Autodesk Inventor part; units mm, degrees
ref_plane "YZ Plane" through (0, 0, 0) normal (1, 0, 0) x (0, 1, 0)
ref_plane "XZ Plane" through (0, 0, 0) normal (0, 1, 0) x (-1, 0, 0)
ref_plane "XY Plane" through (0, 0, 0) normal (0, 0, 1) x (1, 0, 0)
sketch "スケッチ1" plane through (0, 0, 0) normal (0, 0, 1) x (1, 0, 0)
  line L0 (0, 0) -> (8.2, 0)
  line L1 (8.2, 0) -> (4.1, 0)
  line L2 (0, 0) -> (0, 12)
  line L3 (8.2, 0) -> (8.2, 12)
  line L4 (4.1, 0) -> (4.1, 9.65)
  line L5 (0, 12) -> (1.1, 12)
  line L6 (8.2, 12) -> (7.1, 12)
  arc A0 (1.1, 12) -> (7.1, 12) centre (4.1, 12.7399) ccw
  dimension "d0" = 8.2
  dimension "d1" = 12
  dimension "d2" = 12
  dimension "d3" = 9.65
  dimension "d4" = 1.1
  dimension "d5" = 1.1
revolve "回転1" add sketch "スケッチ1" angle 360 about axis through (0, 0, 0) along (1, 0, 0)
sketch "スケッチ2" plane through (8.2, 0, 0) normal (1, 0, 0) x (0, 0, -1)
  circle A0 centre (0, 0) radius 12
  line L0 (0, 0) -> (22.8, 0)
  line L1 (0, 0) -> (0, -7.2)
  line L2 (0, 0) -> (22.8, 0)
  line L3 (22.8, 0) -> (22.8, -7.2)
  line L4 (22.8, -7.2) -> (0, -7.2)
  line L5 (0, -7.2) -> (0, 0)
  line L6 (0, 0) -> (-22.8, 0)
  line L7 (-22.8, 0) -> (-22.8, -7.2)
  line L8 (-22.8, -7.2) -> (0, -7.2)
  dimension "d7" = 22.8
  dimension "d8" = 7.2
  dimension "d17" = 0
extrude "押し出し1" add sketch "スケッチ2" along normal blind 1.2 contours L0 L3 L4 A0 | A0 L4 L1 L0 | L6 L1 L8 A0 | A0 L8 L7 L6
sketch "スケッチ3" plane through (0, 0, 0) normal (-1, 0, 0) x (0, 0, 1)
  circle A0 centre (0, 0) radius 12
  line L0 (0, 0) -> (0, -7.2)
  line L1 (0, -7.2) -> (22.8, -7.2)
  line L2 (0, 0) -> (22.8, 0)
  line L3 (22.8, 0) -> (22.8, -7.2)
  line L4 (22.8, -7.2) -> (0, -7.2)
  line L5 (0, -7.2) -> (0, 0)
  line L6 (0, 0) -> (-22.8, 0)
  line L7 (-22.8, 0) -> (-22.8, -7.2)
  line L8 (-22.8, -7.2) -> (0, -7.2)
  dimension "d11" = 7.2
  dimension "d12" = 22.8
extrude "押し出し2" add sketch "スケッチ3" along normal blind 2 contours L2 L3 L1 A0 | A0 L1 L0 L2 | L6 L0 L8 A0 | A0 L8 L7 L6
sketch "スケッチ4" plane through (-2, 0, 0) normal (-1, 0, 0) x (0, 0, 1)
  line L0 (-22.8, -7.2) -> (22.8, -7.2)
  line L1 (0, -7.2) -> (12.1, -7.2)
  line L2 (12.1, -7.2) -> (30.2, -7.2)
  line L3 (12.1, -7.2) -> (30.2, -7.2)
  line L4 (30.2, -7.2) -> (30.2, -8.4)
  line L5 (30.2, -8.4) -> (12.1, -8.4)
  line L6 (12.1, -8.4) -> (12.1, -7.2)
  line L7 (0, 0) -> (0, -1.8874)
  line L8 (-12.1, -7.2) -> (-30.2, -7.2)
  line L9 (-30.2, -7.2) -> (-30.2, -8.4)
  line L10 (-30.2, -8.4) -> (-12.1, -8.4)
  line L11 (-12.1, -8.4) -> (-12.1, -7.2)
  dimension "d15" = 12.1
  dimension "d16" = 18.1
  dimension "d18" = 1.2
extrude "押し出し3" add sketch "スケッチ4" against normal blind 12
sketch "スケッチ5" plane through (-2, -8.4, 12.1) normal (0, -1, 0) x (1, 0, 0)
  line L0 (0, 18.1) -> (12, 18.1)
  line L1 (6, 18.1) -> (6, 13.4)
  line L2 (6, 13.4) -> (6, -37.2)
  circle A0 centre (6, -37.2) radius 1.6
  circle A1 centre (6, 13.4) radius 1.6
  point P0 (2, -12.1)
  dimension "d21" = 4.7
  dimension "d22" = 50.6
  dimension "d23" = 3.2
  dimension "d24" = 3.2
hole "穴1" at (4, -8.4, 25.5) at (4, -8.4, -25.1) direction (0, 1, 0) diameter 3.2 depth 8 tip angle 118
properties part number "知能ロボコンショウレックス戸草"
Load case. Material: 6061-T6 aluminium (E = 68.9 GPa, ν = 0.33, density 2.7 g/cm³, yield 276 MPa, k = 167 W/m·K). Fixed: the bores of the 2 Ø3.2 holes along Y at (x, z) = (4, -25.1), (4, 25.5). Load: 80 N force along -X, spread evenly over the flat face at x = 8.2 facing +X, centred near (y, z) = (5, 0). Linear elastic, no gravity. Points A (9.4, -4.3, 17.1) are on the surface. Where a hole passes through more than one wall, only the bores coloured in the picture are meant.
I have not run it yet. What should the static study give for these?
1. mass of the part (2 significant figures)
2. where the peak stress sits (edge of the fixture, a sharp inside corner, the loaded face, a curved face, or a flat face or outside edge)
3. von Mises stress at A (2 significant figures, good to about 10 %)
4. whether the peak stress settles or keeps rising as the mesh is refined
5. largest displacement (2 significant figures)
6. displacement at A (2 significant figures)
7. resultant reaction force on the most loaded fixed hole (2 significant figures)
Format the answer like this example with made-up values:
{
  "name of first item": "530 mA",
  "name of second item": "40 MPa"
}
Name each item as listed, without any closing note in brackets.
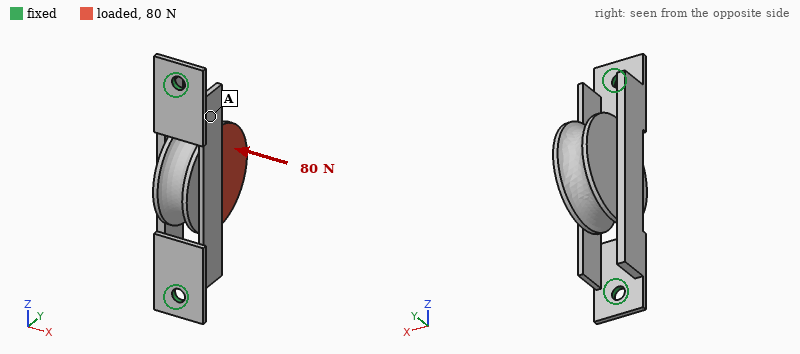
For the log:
{
  "mass of the part": "12 g",
  "where the peak stress sits": "edge of the fixture",
  "von Mises stress at A": "17 MPa",
  "whether the peak stress settles or keeps rising as the mesh is refined": "keeps rising",
  "largest displacement": "0.14 mm",
  "displacement at A": "0.042 mm",
  "resultant reaction force on the most loaded fixed hole": "44 N"
}
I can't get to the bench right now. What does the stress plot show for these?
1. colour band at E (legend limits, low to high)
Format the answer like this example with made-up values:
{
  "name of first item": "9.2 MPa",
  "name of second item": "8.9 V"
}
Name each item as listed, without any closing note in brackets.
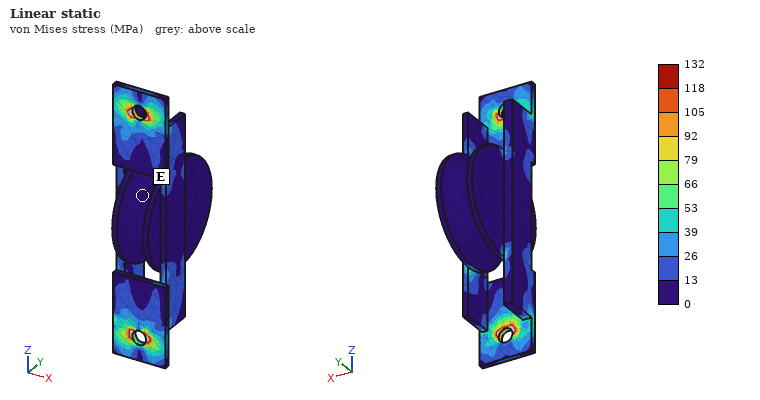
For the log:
{
  "colour band at E": "0 to 13 MPa"
}
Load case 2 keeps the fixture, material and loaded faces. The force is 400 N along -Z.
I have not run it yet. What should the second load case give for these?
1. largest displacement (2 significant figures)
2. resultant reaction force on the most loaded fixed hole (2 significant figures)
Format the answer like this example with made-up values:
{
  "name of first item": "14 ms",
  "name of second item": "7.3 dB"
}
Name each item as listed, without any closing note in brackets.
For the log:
{
  "largest displacement": "22 µm",
  "resultant reaction force on the most loaded fixed hole": "230 N"
}
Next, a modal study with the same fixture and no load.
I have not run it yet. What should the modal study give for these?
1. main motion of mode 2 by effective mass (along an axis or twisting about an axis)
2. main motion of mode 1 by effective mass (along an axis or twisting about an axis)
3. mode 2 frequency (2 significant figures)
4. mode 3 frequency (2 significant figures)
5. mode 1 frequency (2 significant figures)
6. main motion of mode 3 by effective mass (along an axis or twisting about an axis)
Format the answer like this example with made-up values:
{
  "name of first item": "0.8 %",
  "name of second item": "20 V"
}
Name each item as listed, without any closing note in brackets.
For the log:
{
  "main motion of mode 2 by effective mass": "along Y",
  "main motion of mode 1 by effective mass": "along X",
  "mode 2 frequency": "4900 Hz",
  "mode 3 frequency": "8600 Hz",
  "mode 1 frequency": "1900 Hz",
  "main motion of mode 3 by effective mass": "along X"
}
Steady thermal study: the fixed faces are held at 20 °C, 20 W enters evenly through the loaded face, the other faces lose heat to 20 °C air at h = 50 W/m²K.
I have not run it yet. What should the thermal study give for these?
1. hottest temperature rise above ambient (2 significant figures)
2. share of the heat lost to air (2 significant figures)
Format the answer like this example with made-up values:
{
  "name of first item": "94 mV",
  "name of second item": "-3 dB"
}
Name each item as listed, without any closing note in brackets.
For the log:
{
  "hottest temperature rise above ambient": "46 K",
  "share of the heat lost to air": "23 %"
}
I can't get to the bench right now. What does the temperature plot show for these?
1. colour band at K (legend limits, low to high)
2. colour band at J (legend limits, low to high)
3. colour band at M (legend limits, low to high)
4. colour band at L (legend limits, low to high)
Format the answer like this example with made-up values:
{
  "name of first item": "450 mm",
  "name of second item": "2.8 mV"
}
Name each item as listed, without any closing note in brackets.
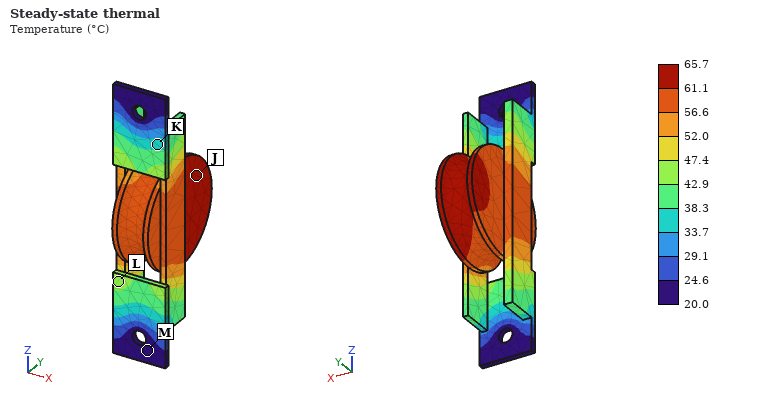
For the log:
{
  "colour band at K": "33.7 to 38.3 °C",
  "colour band at J": "61.1 to 65.7 °C",
  "colour band at M": "20.0 to 24.6 °C",
  "colour band at L": "42.9 to 47.4 °C"
}
